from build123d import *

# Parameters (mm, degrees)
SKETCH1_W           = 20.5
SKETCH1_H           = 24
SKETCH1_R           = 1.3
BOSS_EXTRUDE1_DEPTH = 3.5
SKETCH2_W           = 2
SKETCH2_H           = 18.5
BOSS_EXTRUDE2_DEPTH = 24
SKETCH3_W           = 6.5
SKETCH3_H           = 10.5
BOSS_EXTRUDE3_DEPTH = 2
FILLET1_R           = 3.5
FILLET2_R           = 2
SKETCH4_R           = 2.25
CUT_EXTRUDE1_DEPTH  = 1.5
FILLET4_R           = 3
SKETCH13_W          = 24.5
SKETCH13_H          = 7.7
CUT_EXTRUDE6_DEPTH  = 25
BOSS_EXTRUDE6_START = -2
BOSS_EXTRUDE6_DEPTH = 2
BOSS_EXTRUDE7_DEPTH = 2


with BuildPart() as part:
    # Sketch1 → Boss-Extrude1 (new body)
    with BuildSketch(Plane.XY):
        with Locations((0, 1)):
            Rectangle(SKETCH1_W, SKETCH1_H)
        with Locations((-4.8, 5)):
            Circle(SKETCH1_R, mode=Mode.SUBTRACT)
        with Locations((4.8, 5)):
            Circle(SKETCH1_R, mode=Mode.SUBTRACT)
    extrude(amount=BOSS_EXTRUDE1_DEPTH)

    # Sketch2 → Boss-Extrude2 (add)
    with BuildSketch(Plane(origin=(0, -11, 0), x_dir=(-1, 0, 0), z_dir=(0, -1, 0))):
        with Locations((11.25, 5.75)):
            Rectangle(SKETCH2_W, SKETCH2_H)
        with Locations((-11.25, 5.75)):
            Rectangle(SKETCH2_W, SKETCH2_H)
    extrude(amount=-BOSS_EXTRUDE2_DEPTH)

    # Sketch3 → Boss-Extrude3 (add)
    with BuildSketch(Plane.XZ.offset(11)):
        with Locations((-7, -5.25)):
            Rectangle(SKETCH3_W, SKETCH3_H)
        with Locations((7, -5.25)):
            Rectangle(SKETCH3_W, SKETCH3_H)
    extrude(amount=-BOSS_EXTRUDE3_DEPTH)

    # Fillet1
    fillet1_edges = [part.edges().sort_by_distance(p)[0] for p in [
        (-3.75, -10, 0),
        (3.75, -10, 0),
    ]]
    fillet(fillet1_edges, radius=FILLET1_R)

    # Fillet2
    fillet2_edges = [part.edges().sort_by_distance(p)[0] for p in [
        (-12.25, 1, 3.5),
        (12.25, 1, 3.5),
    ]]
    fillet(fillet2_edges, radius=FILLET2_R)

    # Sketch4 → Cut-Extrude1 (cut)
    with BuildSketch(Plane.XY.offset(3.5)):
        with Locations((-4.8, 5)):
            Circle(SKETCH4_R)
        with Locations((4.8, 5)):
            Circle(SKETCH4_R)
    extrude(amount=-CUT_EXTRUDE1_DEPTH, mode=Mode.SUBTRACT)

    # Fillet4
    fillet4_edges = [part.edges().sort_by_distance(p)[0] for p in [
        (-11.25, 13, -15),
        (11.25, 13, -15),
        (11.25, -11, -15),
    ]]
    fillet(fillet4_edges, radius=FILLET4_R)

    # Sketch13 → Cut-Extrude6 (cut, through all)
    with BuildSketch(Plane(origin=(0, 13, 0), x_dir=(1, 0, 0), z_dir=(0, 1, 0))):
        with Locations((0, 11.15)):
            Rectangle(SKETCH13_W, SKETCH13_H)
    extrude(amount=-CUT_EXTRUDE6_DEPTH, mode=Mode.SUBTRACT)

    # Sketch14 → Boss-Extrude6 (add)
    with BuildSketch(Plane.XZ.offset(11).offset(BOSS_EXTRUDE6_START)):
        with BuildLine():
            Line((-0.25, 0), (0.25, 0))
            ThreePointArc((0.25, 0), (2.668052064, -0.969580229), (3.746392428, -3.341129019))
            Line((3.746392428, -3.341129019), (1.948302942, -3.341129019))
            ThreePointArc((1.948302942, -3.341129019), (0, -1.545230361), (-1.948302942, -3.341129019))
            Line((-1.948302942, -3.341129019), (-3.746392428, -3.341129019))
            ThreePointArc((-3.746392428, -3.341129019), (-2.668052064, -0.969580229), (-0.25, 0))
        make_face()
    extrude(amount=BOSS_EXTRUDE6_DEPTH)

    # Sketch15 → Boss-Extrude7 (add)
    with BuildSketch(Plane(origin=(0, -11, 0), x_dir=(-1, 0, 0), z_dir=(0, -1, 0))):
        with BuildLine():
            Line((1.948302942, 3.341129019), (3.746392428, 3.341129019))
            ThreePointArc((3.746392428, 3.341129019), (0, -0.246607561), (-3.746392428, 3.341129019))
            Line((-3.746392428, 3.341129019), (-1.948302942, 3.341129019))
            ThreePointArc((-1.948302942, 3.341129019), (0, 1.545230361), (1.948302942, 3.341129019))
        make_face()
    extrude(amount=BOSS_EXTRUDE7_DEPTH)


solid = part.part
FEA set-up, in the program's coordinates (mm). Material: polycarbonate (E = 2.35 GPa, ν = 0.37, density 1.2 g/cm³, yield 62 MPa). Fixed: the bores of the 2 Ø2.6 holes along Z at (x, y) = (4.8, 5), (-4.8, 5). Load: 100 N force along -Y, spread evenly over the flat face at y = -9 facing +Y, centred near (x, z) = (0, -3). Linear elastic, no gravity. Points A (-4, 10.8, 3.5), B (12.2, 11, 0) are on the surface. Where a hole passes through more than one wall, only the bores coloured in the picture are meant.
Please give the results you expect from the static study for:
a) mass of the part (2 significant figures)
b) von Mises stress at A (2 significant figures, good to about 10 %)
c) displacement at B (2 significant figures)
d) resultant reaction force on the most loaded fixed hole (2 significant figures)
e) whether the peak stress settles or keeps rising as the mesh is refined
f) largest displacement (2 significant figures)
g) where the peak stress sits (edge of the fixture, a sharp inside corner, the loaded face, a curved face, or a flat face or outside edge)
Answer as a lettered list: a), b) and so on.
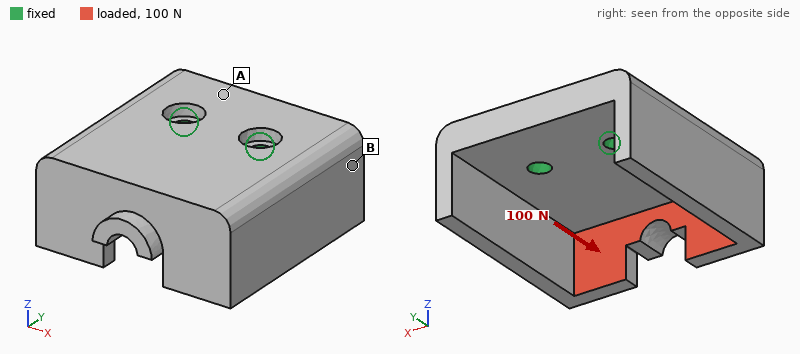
a) 3.5 g
b) 4.5 MPa
c) 0.094 mm
d) 52 N
e) keeps rising
f) 0.37 mm
g) edge of the fixture
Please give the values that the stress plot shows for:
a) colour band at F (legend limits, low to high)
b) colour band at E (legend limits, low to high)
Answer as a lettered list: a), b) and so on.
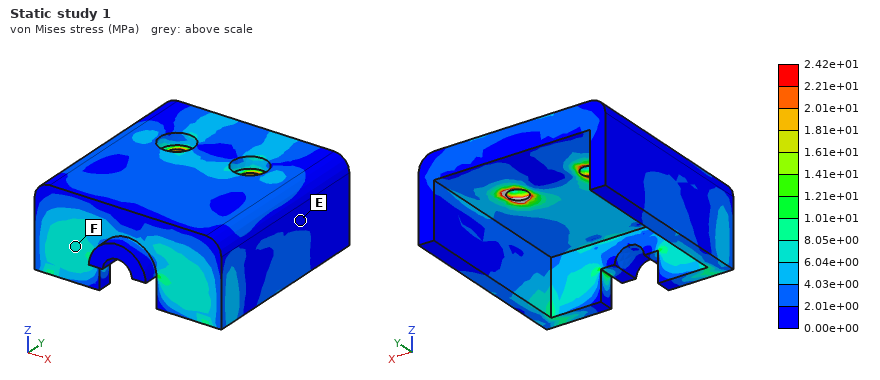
a) 6.04e+00 to 8.05e+00 MPa
b) 0.00e+00 to 2.01e+00 MPa
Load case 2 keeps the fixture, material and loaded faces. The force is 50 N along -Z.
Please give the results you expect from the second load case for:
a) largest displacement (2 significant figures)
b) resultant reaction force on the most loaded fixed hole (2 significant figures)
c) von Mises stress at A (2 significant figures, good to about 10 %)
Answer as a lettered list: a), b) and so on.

a) 0.42 mm
b) 25 N
c) 3.6 MPa
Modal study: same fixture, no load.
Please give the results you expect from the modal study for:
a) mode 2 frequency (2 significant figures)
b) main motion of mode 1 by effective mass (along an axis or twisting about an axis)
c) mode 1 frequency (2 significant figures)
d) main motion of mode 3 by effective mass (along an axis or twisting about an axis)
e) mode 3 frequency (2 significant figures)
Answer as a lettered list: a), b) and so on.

a) 2500 Hz
b) along Z
c) 1600 Hz
d) along Z
e) 4500 Hz
